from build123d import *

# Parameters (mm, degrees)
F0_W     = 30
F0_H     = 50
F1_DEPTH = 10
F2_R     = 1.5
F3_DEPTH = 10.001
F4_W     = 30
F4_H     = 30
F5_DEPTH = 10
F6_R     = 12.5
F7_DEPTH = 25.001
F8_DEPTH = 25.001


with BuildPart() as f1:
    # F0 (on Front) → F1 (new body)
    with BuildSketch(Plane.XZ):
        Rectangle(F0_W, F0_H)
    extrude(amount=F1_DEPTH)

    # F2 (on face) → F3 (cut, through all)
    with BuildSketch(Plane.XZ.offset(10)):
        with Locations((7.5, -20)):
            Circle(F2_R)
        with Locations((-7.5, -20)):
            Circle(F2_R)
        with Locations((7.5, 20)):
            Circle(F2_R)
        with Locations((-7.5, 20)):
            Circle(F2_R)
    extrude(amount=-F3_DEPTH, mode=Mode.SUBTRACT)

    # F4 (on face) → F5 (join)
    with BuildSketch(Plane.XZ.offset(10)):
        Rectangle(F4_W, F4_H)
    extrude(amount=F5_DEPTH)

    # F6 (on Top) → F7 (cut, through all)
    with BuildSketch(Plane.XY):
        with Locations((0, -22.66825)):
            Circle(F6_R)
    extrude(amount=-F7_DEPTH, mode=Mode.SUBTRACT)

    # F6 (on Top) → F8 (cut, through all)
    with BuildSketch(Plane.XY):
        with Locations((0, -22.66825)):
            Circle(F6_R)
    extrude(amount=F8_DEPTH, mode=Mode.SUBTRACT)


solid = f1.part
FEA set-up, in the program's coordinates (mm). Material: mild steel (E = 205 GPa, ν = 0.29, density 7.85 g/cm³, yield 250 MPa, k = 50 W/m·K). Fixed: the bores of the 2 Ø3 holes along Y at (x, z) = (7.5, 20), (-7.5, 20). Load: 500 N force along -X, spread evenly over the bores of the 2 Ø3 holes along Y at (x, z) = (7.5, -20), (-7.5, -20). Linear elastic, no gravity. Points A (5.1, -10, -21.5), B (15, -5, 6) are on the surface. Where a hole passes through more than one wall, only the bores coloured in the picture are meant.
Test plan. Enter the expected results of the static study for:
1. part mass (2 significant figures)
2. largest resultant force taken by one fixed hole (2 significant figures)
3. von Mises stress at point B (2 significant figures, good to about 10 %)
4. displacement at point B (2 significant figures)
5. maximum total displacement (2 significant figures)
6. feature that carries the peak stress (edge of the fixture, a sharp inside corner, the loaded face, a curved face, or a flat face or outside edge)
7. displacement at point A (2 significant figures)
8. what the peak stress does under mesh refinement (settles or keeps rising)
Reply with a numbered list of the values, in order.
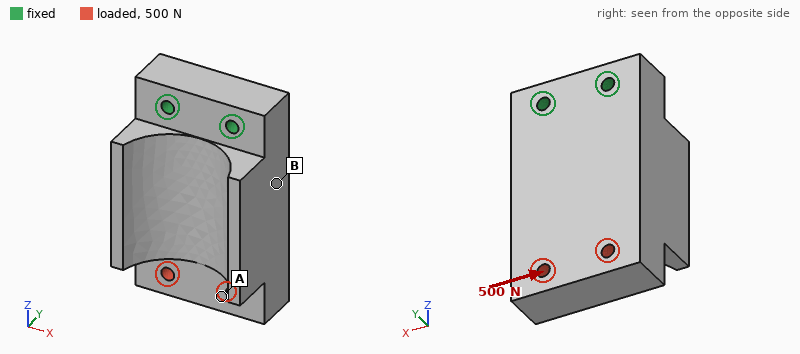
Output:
1. 140 g
2. 1.2 kN
3. 6.8 MPa
4. 1.7 µm
5. 5.0 µm
6. edge of the fixture
7. 4.3 µm
8. keeps rising
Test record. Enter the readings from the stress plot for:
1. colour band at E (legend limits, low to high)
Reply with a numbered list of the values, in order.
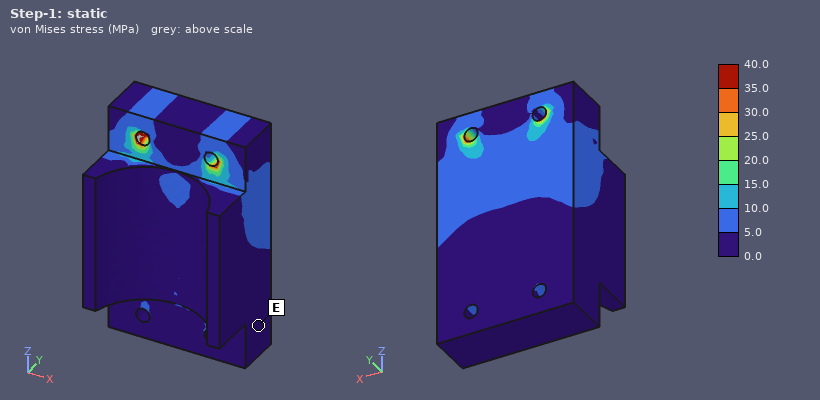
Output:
1. 0.0 to 5.0 MPa
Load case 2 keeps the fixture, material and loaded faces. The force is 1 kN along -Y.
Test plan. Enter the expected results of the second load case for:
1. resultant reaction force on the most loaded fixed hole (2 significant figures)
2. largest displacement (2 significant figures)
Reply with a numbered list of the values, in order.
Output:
1. 510 N
2. 42 µm
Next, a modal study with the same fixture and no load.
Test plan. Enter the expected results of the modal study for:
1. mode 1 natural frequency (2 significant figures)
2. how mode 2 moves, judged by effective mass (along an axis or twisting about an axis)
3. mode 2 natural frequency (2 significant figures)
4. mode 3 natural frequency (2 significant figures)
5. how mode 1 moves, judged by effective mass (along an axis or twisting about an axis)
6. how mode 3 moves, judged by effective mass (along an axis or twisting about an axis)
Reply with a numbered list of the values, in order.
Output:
1. 3800 Hz
2. along X
3. 7600 Hz
4. 9900 Hz
5. along Y
6. twisting about Z
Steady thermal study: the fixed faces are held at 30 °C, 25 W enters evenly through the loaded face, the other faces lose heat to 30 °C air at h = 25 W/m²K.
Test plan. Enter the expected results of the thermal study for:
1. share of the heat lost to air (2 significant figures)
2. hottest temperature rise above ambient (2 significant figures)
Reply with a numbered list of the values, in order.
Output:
1. 15 %
2. 57 K
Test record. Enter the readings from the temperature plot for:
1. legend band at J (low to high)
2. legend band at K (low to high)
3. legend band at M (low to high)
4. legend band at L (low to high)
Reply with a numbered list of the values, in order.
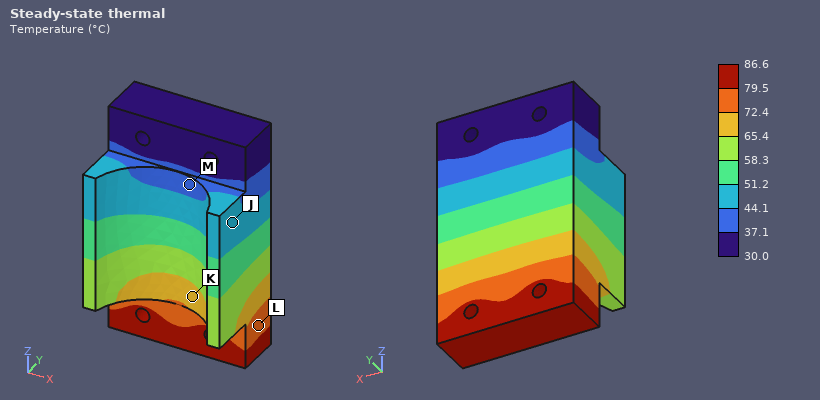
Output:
1. 44.1 to 51.2 °C
2. 65.4 to 72.4 °C
3. 37.1 to 44.1 °C
4. 72.4 to 79.5 °C
